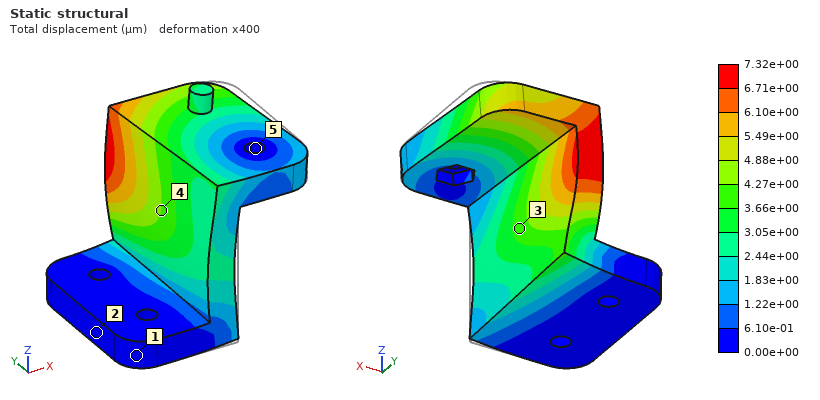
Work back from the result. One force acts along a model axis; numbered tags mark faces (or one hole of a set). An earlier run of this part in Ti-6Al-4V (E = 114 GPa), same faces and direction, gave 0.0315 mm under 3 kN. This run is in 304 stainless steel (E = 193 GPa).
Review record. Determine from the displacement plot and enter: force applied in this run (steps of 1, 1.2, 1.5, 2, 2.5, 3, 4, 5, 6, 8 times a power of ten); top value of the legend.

1.2 kN
7.32e+00 µm
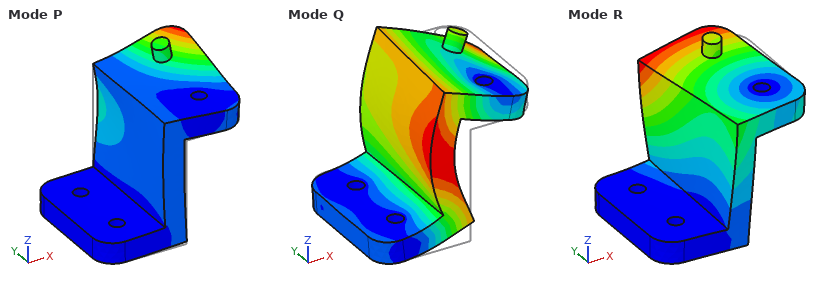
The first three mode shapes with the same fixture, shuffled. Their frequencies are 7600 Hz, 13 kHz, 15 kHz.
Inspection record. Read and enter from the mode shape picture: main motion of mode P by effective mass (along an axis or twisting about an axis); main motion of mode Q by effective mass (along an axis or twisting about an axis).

along Z
along Z
